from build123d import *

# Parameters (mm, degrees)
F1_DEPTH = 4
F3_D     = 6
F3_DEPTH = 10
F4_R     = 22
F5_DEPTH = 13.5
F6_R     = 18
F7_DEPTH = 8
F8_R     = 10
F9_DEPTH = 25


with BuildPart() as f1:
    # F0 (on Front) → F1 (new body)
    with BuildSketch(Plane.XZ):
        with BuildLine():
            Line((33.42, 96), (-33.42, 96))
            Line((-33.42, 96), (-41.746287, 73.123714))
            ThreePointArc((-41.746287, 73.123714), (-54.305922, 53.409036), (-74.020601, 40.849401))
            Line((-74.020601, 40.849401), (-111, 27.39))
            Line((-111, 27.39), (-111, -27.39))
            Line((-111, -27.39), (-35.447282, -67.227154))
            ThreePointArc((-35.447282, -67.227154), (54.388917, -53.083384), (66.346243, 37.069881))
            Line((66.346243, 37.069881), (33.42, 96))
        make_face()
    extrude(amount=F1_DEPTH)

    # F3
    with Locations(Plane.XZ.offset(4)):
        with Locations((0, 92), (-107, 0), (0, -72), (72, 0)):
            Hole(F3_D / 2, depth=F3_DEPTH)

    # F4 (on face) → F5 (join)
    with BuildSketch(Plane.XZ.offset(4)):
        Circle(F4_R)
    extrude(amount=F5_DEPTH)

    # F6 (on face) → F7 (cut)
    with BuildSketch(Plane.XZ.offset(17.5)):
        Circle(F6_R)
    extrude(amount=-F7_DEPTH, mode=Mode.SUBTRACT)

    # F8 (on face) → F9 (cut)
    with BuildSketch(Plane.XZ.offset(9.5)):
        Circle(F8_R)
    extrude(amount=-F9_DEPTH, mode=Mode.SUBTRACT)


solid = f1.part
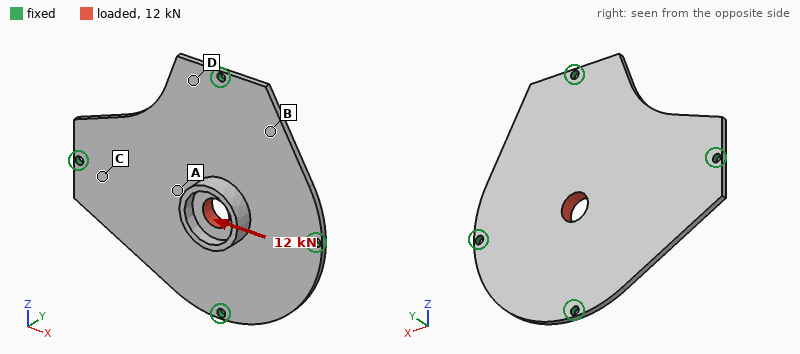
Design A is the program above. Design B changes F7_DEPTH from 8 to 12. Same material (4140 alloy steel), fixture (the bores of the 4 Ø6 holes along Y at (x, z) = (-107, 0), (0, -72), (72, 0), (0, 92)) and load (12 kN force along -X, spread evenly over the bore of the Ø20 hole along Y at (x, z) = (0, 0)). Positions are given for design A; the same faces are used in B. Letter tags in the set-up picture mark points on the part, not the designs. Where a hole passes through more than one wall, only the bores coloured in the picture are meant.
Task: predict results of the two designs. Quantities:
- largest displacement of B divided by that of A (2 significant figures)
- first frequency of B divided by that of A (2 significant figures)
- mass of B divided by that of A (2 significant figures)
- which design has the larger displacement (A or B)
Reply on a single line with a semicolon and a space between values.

0.34; 1.0; 0.97; A
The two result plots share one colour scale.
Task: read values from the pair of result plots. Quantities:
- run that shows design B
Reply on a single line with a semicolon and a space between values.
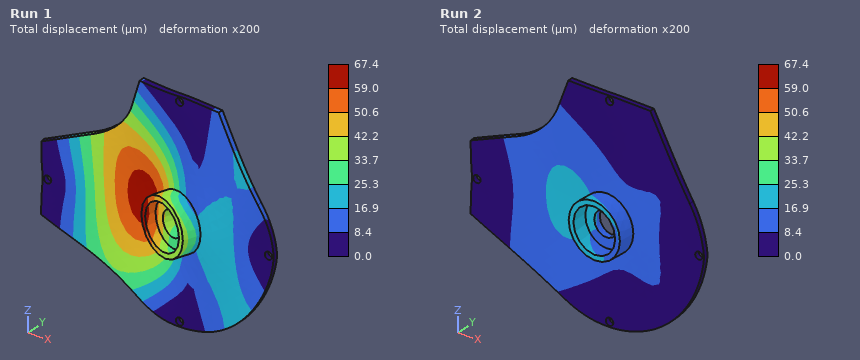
Run 2
